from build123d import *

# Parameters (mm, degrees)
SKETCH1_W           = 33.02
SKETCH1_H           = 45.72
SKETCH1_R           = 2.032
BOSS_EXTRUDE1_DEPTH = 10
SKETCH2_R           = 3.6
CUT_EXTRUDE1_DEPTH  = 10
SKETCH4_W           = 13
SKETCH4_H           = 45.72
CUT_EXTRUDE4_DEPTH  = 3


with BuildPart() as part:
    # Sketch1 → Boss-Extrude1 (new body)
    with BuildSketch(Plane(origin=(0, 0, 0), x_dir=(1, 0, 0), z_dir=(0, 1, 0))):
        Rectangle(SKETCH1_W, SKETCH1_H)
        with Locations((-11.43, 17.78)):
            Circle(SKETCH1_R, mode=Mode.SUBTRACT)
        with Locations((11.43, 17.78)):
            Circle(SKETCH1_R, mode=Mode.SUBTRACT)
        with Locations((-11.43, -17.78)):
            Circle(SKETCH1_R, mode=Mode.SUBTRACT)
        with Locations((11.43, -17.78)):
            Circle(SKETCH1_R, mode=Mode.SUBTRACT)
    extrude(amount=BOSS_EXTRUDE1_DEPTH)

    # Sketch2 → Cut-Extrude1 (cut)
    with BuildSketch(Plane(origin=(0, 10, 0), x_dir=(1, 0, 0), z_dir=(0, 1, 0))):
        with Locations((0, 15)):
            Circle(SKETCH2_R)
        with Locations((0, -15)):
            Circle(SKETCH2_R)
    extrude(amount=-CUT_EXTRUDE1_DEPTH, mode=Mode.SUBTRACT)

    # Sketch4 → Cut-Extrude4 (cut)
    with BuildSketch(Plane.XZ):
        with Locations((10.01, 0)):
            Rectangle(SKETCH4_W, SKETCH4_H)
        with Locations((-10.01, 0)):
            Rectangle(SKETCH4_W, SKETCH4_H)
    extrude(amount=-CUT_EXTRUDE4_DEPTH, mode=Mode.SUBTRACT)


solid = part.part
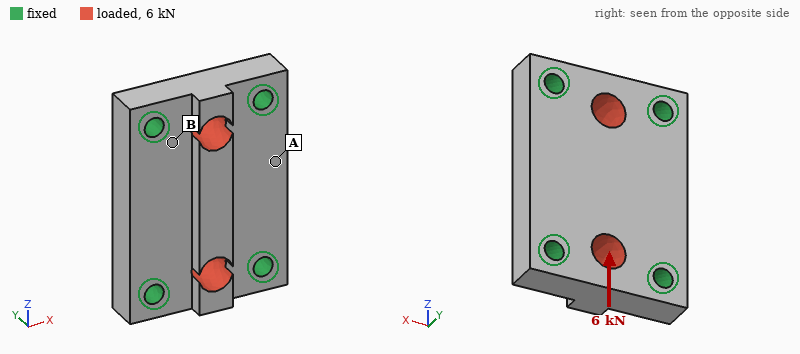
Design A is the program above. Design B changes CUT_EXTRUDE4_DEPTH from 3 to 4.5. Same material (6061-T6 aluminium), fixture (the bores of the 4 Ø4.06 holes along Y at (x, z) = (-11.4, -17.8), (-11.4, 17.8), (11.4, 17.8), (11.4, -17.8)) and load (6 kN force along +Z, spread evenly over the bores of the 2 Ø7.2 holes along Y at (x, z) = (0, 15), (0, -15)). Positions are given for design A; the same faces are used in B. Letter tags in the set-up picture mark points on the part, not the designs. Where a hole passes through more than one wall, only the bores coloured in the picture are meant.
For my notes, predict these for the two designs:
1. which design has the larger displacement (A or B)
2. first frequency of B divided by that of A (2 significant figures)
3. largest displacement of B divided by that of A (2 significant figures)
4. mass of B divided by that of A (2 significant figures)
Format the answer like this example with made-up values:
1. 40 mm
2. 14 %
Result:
1. B
2. 0.86
3. 1.8
4. 0.84
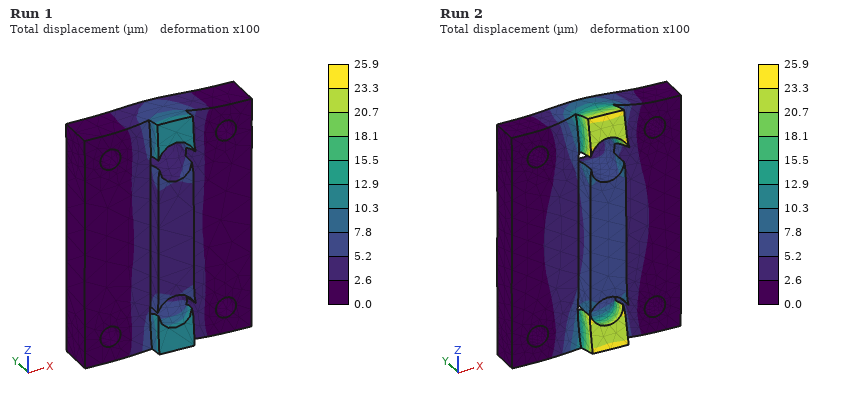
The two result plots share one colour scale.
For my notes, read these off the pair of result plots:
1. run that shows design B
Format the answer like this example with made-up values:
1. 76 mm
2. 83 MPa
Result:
1. Run 2
